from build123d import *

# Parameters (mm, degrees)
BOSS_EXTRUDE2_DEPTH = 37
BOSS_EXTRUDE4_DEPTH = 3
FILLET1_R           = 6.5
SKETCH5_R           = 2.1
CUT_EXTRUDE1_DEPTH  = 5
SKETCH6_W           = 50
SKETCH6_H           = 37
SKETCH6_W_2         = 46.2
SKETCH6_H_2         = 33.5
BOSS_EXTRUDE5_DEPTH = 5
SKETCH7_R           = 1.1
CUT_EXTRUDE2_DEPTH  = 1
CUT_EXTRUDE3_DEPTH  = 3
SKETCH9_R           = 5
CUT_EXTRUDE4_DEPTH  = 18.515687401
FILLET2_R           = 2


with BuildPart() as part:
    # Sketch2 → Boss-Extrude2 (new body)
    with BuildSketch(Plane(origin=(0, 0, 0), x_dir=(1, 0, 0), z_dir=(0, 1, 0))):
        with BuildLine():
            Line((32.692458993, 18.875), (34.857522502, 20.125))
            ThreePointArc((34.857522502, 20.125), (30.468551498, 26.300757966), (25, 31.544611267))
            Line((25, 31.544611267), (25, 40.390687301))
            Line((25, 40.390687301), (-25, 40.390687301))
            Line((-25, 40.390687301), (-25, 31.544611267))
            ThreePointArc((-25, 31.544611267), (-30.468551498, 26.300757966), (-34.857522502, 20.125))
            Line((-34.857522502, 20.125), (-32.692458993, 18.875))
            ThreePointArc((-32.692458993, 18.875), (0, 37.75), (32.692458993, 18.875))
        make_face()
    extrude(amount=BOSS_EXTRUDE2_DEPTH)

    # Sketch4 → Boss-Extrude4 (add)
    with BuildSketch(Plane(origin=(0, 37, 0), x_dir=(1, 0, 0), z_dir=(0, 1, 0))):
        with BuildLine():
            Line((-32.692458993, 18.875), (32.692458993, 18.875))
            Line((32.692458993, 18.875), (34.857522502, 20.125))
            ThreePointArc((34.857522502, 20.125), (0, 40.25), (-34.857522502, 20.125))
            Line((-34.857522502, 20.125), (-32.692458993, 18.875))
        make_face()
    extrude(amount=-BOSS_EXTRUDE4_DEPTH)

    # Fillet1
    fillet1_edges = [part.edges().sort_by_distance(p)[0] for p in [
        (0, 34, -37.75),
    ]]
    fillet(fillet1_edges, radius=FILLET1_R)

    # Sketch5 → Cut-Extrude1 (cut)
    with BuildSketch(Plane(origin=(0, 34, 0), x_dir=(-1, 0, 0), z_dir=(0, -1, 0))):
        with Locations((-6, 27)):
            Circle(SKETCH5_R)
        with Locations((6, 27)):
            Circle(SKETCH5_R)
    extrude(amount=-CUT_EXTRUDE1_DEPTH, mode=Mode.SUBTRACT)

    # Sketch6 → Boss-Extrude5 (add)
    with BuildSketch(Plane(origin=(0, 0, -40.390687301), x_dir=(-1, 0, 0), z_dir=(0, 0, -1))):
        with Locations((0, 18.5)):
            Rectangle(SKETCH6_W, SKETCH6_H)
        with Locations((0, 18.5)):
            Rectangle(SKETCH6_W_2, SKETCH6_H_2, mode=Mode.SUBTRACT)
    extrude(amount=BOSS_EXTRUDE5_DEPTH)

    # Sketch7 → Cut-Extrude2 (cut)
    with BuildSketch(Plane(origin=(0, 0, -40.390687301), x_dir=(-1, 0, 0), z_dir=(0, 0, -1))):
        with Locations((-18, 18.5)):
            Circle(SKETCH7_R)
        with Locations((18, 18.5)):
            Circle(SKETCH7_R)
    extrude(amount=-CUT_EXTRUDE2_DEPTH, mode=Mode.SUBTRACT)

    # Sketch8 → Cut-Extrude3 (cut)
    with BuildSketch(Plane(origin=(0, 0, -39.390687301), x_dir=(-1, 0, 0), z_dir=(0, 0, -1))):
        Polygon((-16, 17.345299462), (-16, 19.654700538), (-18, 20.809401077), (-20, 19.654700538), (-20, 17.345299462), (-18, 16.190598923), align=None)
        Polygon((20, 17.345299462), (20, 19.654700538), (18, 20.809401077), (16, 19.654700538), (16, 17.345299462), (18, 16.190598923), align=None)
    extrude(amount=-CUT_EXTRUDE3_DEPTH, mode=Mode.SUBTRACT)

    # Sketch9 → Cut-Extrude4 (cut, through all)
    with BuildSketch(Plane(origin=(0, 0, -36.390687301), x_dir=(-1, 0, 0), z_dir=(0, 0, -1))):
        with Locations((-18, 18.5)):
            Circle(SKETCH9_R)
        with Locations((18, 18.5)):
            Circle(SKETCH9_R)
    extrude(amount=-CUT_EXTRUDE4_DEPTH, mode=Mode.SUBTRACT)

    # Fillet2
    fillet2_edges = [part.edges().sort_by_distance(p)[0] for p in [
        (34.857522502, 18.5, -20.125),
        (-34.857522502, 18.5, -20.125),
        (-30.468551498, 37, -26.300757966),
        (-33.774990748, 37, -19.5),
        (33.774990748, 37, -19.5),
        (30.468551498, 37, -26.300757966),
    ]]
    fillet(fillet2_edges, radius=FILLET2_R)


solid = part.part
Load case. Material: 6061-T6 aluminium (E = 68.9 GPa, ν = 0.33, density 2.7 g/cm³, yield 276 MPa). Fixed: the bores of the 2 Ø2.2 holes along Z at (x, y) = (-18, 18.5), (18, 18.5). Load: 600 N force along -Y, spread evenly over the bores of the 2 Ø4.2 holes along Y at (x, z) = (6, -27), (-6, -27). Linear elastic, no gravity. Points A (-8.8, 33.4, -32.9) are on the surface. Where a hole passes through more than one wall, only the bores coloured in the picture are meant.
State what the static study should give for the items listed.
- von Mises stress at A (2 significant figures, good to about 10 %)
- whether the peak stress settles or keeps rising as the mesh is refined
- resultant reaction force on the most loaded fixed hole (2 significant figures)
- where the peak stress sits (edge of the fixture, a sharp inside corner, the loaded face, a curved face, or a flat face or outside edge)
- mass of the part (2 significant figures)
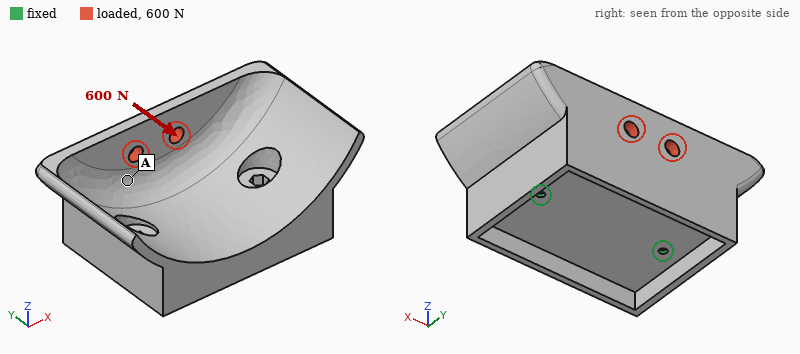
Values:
42 MPa
keeps rising
310 N
edge of the fixture
46 g
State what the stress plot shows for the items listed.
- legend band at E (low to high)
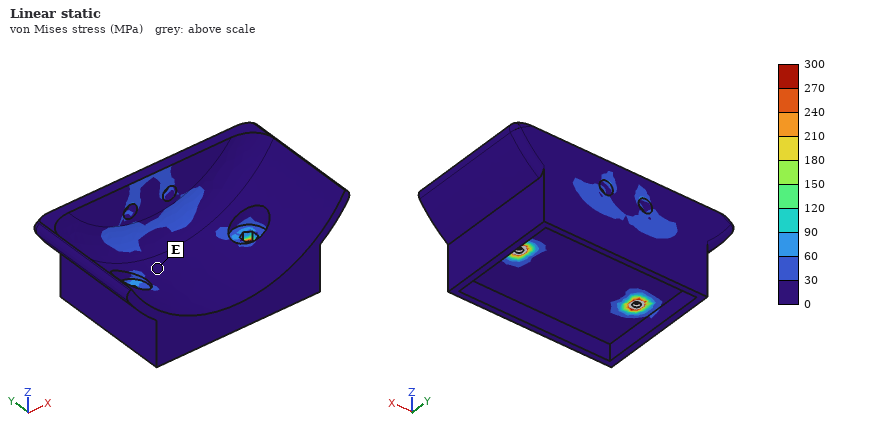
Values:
0 to 30 MPa
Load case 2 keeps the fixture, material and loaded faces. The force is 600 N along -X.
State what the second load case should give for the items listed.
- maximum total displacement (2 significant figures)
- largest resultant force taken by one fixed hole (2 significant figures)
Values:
37 µm
460 N
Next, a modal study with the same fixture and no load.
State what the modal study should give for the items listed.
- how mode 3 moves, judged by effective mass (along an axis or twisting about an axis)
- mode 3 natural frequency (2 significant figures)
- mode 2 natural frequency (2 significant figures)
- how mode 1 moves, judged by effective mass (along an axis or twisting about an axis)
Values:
along X
6100 Hz
3900 Hz
along Y
